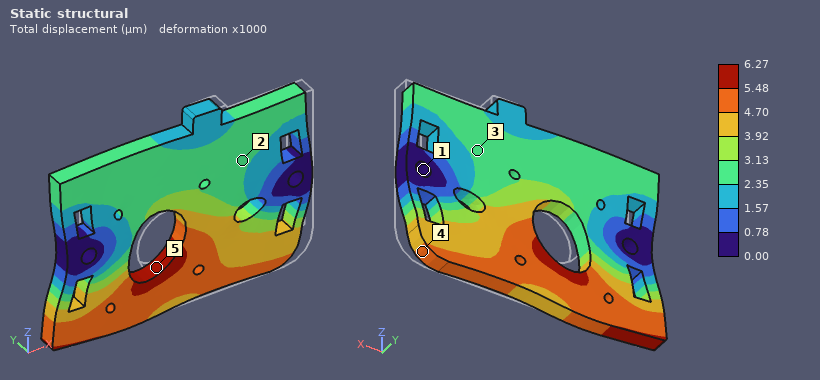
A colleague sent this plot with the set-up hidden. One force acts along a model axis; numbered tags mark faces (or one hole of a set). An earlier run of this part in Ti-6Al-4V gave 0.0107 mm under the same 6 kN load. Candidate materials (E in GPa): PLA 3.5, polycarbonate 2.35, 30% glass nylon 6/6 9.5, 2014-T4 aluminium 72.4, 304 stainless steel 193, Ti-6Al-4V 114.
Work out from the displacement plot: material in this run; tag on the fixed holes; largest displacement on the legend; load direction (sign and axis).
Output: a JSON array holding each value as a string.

["304 stainless steel", "1", "6.27 µm", "-X"]
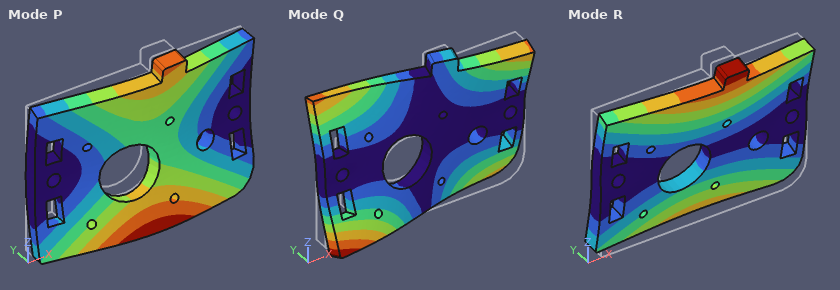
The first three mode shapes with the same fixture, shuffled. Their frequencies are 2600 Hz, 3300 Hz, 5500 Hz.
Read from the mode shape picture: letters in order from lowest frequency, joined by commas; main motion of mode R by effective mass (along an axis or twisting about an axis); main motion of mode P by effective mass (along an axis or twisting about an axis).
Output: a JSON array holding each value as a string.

["R, P, Q", "twisting about X", "along Y"]
